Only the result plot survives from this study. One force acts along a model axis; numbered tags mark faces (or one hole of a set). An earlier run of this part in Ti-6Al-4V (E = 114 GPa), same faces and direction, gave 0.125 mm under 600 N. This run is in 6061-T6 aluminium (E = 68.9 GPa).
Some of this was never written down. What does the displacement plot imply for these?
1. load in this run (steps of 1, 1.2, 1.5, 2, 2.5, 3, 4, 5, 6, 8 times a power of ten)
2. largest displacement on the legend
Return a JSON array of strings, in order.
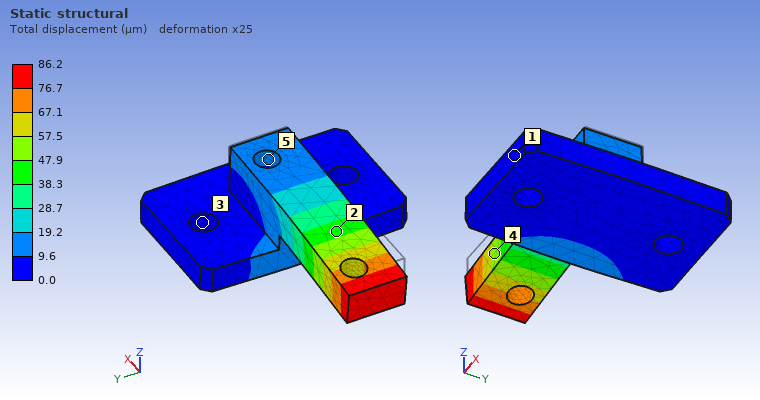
["250 N", "86.2 µm"]
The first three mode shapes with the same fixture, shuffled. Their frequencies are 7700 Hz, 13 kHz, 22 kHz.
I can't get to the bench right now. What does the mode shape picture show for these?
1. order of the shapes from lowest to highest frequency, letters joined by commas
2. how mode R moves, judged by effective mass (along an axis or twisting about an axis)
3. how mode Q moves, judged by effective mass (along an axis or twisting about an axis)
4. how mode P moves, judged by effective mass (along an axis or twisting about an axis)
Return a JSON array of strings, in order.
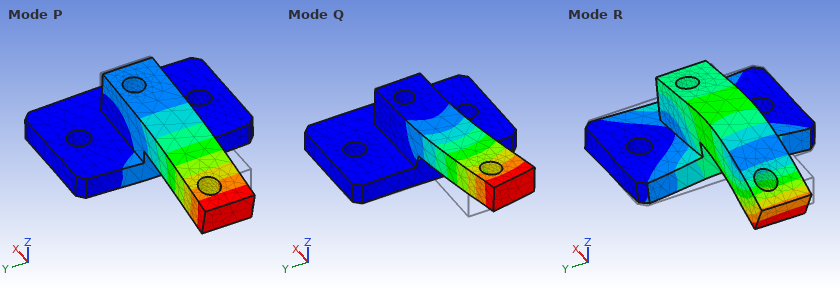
["P, Q, R", "along X", "along Y", "along Z"]
